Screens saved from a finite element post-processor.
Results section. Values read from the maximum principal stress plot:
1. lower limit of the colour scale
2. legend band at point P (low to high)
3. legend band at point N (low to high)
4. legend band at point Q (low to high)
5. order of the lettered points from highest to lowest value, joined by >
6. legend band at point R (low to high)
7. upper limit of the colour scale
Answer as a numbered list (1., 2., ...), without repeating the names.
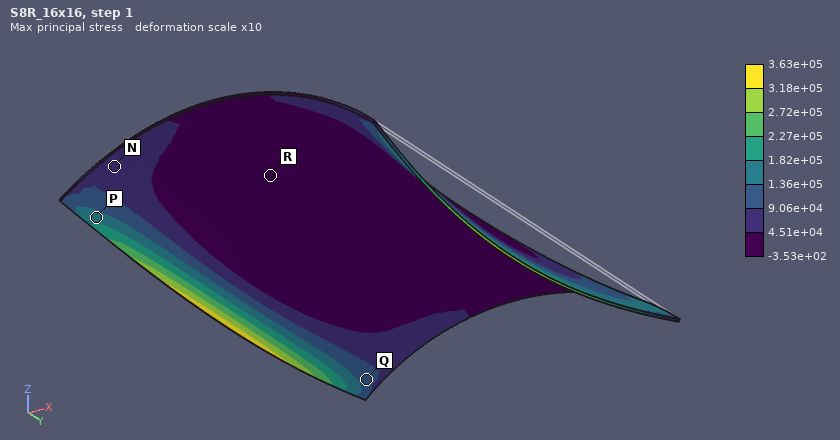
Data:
1. -3.53e+02
2. 1.36e+05 to 1.82e+05
3. 4.51e+04 to 9.06e+04
4. 9.06e+04 to 1.36e+05
5. P > Q > N > R
6. -3.53e+02 to 4.51e+04
7. 3.63e+05
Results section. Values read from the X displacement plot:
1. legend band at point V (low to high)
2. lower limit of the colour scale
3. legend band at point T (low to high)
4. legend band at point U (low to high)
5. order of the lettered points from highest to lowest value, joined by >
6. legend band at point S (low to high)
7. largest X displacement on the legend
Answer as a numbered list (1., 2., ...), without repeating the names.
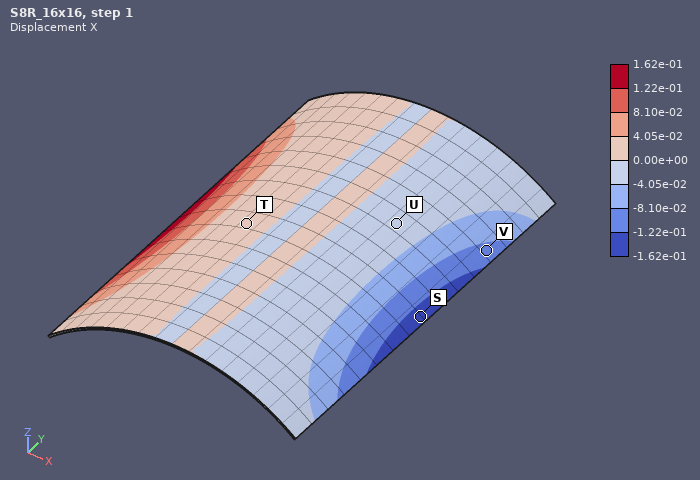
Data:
1. -1.22e-01 to -8.10e-02
2. -1.62e-01
3. 0.00e+00 to 4.05e-02
4. -4.05e-02 to 0.00e+00
5. T > U > V > S
6. -1.62e-01 to -1.22e-01
7. 1.62e-01
